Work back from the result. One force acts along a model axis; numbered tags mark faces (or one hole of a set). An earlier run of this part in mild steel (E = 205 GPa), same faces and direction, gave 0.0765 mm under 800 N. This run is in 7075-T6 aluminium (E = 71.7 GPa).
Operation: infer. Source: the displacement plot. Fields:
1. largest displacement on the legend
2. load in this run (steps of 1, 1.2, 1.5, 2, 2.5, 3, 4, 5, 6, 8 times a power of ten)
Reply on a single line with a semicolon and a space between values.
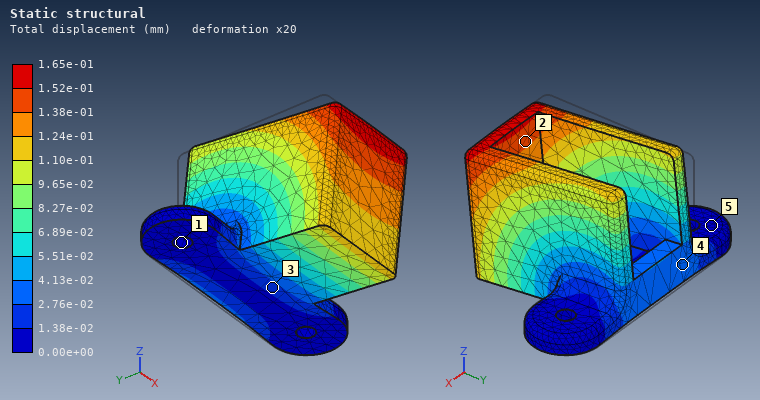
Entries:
1.65e-01 mm; 600 N
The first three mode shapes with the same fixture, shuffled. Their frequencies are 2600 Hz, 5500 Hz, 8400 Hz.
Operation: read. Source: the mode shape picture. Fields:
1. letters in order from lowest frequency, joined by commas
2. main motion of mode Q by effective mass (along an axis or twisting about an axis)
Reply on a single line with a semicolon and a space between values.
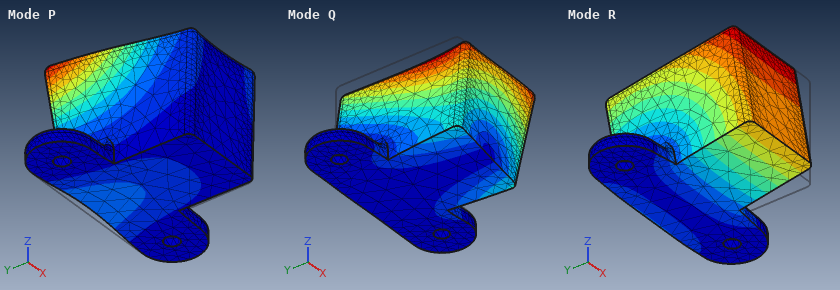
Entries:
R, Q, P; along X
